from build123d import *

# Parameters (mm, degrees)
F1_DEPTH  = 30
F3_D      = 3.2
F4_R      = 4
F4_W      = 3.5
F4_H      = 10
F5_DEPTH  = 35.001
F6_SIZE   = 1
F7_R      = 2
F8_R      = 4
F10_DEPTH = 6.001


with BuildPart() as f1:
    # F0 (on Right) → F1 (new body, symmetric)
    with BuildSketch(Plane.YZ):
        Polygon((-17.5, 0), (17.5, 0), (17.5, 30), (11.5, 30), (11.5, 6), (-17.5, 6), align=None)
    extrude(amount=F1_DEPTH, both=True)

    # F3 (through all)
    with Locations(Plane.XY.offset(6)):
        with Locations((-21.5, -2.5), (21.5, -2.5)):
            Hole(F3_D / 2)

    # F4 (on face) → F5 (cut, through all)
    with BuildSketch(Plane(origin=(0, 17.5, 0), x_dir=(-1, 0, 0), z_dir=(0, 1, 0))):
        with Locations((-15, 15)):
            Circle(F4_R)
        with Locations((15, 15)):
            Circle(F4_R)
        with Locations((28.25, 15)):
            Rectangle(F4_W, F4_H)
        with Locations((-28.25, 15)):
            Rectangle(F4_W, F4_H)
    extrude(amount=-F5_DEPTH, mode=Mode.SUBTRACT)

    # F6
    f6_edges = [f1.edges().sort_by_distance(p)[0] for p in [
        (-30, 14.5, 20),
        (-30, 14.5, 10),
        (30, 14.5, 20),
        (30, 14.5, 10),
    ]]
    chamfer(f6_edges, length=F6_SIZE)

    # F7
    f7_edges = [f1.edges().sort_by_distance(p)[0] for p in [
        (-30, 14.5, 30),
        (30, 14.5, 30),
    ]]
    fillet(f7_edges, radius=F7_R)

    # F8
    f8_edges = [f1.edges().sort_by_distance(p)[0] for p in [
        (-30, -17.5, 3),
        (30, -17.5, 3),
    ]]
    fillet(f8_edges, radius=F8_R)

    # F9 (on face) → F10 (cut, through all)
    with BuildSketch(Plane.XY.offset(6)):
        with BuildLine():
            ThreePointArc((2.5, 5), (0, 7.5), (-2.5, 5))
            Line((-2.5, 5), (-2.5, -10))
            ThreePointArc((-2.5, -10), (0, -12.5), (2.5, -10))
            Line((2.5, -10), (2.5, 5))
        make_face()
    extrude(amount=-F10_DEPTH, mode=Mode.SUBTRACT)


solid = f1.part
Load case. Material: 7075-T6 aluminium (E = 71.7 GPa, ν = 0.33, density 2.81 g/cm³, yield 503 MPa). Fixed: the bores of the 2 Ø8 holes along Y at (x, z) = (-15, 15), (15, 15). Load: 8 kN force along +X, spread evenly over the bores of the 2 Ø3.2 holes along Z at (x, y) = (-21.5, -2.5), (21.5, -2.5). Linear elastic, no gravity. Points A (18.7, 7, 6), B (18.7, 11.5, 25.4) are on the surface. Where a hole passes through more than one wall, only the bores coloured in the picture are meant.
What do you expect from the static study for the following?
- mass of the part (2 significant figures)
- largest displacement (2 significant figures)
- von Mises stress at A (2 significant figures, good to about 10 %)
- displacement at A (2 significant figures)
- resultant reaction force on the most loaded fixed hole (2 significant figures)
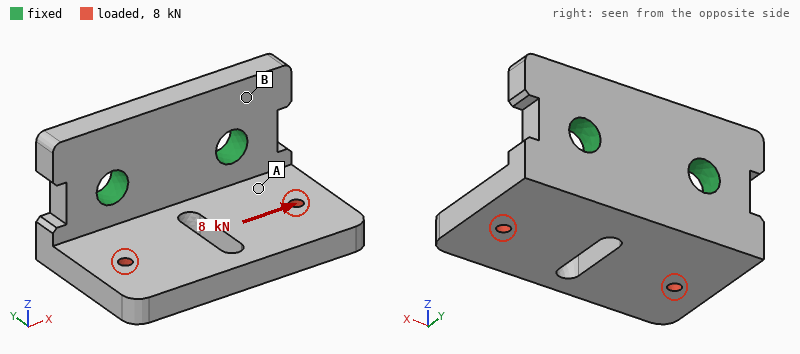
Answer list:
55 g
0.16 mm
88 MPa
0.055 mm
5.9 kN
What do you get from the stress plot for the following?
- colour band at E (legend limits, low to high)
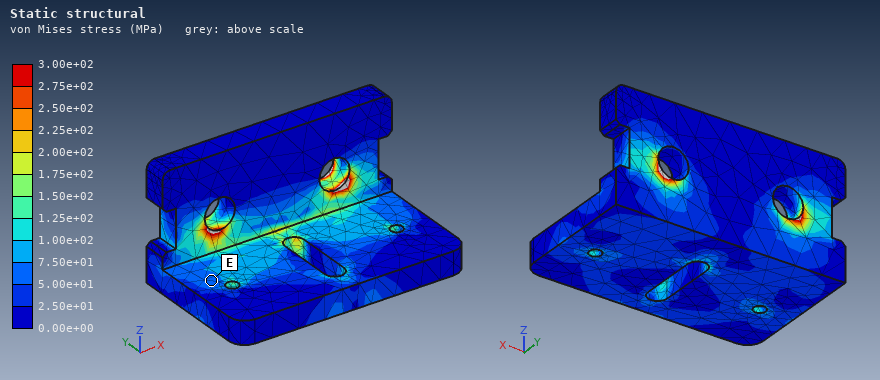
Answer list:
5.00e+01 to 7.50e+01 MPa
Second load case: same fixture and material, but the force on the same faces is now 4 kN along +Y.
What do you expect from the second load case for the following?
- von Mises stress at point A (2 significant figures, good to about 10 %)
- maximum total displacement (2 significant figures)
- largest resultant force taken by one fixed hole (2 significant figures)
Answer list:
24 MPa
0.11 mm
2.0 kN
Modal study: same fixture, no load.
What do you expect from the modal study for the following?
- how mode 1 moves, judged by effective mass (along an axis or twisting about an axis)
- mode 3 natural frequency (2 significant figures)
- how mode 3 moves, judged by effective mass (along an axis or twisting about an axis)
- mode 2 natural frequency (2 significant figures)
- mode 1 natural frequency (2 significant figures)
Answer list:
along Z
8700 Hz
along X
5400 Hz
3300 Hz
